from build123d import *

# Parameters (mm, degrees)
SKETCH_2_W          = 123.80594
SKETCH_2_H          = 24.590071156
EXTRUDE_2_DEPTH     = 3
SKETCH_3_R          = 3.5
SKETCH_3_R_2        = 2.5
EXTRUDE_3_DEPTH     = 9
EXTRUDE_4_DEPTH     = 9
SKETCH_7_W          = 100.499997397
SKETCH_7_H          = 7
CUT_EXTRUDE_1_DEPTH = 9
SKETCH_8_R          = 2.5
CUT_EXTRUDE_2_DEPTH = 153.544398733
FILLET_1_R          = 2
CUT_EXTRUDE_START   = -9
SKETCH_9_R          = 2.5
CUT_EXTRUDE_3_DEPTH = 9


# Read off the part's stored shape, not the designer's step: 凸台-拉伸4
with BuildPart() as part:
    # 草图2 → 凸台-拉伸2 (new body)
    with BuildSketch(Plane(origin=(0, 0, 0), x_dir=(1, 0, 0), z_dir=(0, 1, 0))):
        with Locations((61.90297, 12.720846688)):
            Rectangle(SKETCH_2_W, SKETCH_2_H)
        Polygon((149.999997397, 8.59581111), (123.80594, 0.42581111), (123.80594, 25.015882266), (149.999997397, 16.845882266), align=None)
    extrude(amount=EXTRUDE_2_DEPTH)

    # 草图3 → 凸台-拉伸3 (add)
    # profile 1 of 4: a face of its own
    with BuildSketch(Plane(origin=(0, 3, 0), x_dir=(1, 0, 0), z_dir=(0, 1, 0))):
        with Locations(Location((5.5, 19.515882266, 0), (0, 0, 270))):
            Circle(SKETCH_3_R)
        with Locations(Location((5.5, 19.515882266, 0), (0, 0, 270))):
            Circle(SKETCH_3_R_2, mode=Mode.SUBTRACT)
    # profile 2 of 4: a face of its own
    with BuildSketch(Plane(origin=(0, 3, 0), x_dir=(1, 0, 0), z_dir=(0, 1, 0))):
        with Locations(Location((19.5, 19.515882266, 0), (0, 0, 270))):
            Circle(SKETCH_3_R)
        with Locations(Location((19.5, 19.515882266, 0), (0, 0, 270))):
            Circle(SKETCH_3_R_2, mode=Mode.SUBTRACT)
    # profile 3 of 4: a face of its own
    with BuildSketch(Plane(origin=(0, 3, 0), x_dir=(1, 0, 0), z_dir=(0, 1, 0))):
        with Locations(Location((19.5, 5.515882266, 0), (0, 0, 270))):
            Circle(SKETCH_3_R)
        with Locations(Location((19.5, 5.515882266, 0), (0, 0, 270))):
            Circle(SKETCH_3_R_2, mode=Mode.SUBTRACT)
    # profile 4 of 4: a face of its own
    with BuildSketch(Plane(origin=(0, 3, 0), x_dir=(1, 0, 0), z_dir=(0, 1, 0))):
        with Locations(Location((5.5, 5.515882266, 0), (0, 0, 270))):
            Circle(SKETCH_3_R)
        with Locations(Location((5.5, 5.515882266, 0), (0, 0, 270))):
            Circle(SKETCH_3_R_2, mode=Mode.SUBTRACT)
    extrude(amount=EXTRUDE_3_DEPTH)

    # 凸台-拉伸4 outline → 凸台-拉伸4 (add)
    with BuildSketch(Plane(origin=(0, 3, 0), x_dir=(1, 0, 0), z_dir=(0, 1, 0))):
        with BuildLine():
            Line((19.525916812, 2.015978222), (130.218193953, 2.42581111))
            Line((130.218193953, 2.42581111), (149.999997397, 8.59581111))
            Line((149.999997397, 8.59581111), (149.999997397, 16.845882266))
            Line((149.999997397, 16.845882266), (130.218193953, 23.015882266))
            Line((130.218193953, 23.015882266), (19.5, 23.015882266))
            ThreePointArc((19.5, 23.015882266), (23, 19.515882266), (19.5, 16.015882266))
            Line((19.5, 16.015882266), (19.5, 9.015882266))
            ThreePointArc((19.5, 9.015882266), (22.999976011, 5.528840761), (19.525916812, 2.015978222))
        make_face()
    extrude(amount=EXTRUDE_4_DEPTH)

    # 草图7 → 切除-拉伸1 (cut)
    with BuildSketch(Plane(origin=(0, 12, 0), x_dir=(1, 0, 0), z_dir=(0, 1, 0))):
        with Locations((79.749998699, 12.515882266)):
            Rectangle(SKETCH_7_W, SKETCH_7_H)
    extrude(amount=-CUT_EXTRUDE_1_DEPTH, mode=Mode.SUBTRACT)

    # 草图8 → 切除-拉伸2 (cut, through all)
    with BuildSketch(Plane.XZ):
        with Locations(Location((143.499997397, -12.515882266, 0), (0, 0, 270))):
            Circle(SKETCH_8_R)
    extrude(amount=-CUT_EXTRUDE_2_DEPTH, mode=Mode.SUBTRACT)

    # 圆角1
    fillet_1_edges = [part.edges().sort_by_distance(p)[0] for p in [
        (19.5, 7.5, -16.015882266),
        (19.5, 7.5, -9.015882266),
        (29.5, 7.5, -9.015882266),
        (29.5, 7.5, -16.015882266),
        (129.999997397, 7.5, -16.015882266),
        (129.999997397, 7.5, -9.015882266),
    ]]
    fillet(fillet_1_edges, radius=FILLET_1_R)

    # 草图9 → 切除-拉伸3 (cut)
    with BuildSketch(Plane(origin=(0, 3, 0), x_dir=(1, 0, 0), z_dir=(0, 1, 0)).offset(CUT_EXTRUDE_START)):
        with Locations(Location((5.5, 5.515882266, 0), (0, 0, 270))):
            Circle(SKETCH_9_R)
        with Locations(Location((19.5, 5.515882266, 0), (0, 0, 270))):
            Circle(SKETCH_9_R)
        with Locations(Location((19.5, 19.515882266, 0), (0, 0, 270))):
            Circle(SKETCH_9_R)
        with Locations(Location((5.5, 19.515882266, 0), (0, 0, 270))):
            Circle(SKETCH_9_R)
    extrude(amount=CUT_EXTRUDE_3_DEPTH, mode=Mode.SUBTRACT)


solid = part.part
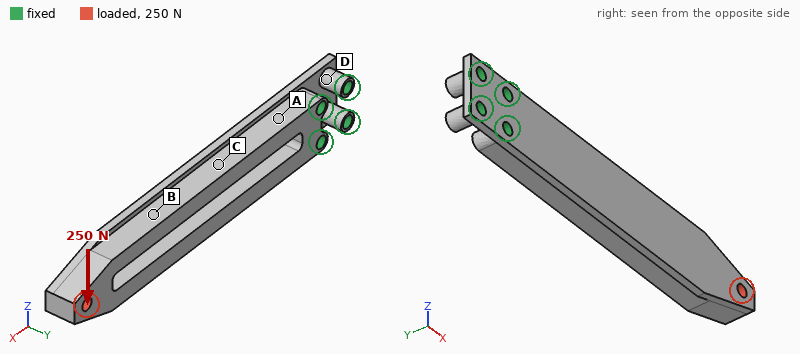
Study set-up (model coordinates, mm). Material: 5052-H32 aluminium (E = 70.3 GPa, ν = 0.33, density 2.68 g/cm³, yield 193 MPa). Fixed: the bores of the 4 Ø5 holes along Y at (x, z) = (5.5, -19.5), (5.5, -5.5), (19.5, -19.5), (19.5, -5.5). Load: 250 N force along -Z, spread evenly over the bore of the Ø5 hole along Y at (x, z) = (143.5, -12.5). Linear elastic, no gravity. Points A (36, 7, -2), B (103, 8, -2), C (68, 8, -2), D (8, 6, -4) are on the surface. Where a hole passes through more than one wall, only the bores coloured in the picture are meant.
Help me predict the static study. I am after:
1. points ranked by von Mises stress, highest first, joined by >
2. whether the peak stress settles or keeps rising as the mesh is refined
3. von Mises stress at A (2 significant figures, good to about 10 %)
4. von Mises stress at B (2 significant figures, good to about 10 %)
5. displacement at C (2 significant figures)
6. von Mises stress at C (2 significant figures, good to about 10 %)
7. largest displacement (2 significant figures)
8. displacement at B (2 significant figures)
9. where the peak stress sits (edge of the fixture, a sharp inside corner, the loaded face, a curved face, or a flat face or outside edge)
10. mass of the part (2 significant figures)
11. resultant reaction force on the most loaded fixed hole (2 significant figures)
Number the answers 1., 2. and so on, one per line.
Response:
1. A > C > B > D
2. keeps rising
3. 29 MPa
4. 12 MPa
5. 0.057 mm
6. 21 MPa
7. 0.28 mm
8. 0.14 mm
9. edge of the fixture
10. 73 g
11. 1.9 kN
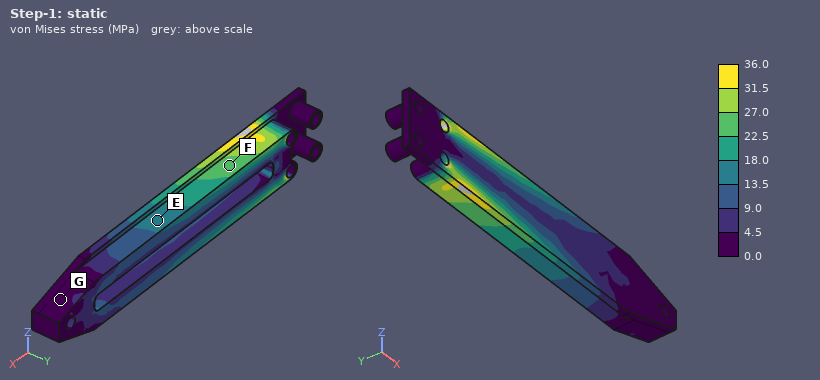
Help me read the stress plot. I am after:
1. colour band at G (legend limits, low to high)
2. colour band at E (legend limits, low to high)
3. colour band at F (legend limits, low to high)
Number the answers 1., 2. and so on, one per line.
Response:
1. 0.0 to 4.5 MPa
2. 13.5 to 18.0 MPa
3. 22.5 to 27.0 MPa
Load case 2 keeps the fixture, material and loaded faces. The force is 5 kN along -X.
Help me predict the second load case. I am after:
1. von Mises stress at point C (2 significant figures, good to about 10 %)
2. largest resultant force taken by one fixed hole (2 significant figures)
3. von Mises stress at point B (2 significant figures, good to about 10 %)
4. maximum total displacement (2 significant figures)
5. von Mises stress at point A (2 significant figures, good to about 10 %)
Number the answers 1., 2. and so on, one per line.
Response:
1. 29 MPa
2. 2.5 kN
3. 30 MPa
4. 0.17 mm
5. 26 MPa
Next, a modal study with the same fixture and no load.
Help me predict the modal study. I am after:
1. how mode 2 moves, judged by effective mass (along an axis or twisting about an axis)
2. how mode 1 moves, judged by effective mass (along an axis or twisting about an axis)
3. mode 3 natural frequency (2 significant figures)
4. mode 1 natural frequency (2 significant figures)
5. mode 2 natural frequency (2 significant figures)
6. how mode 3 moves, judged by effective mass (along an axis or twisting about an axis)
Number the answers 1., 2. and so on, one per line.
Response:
1. along Z
2. along Y
3. 3200 Hz
4. 660 Hz
5. 1200 Hz
6. twisting about X
